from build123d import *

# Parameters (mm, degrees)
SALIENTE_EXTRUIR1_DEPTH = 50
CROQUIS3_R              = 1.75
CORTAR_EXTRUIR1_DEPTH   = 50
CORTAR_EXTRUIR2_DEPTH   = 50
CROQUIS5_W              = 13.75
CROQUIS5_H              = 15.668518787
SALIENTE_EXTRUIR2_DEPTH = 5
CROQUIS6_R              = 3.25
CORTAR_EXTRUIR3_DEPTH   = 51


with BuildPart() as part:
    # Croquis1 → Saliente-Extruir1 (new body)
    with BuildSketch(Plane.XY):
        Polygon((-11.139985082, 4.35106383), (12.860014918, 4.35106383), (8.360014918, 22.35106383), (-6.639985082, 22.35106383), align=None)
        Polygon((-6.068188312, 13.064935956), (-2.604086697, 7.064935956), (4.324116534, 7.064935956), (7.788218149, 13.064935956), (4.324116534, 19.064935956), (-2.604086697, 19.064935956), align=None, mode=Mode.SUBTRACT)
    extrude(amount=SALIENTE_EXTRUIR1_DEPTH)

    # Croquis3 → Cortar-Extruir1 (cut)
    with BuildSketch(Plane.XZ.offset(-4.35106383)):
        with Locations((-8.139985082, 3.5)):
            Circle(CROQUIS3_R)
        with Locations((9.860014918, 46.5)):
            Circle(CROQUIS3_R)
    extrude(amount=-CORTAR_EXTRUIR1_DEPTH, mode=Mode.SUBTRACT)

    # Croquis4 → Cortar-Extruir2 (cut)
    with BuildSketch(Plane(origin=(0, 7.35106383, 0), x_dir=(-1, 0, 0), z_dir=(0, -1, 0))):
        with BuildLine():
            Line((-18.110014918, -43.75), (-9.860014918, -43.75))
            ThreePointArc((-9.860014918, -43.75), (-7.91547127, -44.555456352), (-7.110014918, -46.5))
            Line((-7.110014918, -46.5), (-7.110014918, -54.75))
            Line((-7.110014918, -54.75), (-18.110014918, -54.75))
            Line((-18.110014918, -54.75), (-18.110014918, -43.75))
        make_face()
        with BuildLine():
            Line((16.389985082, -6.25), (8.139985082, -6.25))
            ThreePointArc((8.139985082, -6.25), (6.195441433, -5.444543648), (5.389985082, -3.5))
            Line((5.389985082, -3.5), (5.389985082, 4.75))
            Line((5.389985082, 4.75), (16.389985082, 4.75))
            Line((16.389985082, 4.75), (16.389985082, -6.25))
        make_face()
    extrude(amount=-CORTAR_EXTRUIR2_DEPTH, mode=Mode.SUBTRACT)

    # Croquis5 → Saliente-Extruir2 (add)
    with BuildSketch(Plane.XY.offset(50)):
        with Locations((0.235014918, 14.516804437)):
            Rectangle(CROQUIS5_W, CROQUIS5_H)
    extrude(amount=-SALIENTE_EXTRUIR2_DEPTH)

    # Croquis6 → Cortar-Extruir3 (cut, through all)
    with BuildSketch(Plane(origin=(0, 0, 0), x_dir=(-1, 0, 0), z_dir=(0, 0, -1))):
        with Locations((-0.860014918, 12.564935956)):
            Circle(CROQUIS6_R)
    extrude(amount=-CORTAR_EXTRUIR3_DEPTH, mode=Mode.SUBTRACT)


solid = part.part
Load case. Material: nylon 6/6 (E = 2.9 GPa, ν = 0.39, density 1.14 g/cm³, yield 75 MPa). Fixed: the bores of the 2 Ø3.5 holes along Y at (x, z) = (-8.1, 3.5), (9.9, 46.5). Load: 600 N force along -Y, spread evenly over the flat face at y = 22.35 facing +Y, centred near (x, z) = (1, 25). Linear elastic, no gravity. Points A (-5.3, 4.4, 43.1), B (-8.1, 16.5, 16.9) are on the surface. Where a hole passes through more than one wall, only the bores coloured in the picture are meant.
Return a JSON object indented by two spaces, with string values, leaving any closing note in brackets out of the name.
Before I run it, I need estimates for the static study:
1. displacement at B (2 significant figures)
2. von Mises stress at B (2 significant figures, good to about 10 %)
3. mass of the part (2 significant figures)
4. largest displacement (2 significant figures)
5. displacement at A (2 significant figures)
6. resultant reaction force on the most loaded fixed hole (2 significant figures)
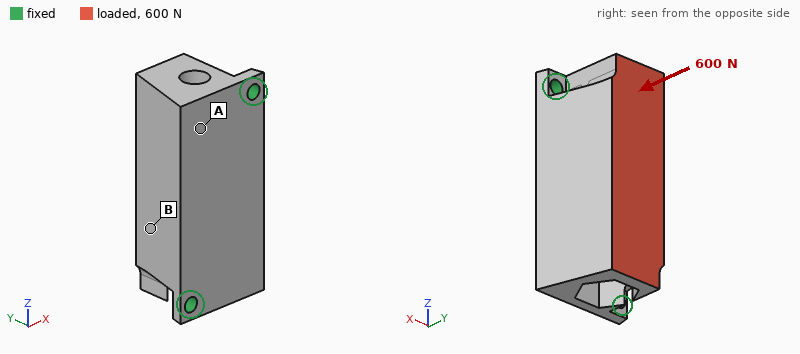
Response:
{
  "displacement at B": "0.079 mm",
  "von Mises stress at B": "7.6 MPa",
  "mass of the part": "13 g",
  "largest displacement": "0.23 mm",
  "displacement at A": "0.051 mm",
  "resultant reaction force on the most loaded fixed hole": "340 N"
}
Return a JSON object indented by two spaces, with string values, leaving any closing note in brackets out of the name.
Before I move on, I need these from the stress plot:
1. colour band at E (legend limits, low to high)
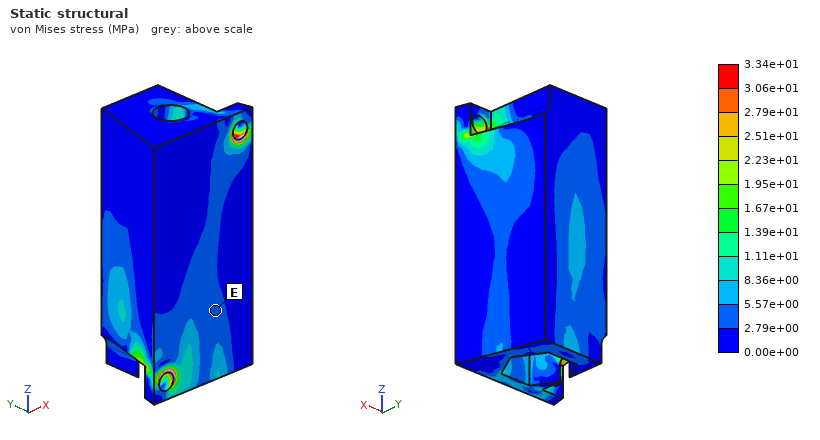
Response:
{
  "colour band at E": "2.79e+00 to 5.57e+00 MPa"
}
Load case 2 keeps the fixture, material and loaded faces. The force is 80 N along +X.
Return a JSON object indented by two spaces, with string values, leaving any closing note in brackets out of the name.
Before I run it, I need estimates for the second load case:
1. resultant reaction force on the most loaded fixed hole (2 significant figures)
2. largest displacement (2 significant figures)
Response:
{
  "resultant reaction force on the most loaded fixed hole": "45 N",
  "largest displacement": "0.38 mm"
}
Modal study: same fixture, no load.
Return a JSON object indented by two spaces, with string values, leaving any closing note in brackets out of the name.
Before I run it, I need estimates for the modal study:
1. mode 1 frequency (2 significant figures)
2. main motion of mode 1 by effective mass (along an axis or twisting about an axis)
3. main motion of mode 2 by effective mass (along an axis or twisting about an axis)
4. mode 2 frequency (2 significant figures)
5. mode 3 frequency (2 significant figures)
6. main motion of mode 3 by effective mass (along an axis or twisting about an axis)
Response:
{
  "mode 1 frequency": "1000 Hz",
  "main motion of mode 1 by effective mass": "along X",
  "main motion of mode 2 by effective mass": "along Y",
  "mode 2 frequency": "3300 Hz",
  "mode 3 frequency": "4500 Hz",
  "main motion of mode 3 by effective mass": "along X"
}
